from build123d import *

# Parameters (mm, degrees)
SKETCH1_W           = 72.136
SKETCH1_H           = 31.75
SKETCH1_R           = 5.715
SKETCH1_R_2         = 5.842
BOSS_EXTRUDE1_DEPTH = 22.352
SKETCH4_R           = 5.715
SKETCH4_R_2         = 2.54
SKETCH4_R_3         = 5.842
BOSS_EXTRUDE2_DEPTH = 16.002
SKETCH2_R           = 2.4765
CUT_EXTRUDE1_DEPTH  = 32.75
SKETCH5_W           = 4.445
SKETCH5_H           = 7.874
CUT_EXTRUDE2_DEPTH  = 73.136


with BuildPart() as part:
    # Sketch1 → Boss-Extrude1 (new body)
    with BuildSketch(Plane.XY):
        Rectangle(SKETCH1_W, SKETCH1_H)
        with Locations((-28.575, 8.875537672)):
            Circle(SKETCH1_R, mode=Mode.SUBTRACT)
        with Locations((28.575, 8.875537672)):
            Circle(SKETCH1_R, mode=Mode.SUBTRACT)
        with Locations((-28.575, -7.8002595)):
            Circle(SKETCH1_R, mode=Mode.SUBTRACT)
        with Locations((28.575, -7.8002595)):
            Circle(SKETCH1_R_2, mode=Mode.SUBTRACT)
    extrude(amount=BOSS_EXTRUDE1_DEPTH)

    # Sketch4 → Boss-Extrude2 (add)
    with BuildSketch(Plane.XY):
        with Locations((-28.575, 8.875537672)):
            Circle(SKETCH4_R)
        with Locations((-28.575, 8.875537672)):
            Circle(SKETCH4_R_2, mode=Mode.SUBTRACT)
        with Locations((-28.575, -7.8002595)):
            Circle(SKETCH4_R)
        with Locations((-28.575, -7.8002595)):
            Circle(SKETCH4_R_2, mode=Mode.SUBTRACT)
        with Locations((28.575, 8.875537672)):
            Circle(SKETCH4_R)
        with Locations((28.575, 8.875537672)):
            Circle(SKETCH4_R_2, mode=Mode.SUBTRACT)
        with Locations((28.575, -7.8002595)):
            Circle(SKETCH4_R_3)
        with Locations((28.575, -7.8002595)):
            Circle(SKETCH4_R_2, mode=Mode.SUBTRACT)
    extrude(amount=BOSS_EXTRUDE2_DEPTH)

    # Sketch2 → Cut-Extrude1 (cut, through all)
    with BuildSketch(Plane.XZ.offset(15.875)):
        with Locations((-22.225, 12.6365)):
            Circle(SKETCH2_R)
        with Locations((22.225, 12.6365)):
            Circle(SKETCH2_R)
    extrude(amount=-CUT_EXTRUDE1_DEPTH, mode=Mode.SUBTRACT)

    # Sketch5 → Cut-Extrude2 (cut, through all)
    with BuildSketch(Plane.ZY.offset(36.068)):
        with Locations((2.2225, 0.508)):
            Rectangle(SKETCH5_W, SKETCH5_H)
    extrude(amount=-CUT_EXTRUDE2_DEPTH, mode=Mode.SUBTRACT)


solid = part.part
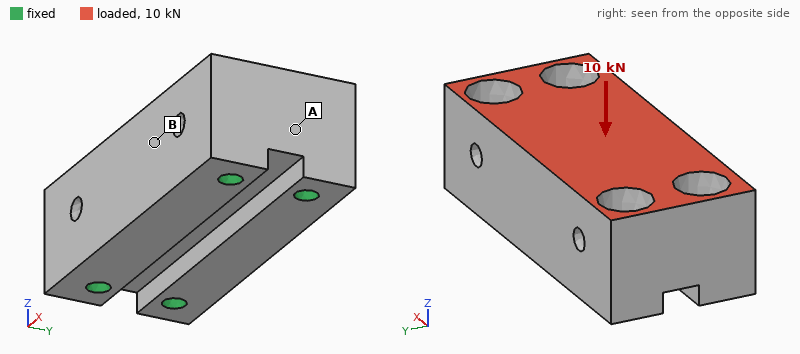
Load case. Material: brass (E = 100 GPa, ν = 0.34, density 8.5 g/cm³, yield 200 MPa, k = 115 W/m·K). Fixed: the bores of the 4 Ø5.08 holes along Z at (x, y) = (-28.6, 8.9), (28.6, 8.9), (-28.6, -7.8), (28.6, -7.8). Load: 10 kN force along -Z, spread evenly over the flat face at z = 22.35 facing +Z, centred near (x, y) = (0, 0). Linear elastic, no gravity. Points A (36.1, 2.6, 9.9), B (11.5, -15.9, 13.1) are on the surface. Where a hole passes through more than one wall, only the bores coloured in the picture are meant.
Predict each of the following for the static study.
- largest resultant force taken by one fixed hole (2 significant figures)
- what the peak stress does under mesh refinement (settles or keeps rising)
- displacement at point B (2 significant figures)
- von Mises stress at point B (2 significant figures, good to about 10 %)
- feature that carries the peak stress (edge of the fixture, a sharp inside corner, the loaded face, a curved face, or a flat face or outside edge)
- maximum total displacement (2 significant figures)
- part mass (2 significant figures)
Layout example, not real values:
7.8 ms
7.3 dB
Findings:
2.8 kN
keeps rising
5.9 µm
11 MPa
edge of the fixture
7.4 µm
370 g
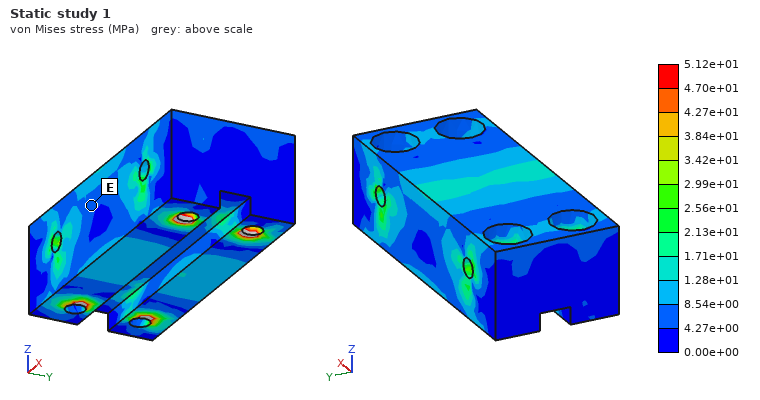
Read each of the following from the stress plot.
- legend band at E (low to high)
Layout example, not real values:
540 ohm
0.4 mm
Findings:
4.27e+00 to 8.54e+00 MPa
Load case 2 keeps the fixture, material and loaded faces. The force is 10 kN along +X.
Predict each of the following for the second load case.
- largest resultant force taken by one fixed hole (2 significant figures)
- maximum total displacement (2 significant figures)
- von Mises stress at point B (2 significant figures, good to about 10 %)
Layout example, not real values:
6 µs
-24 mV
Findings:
2.8 kN
5.7 µm
8.1 MPa
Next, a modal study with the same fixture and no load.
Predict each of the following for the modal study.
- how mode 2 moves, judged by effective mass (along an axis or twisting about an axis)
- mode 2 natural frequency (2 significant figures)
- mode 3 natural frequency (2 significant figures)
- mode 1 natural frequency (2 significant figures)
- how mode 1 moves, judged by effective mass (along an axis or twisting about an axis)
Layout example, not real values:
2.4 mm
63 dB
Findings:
along Y
12 kHz
13 kHz
11 kHz
along Z
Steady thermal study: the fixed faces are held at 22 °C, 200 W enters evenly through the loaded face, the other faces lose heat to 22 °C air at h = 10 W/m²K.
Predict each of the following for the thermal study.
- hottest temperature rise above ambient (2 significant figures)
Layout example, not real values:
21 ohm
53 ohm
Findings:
32 K
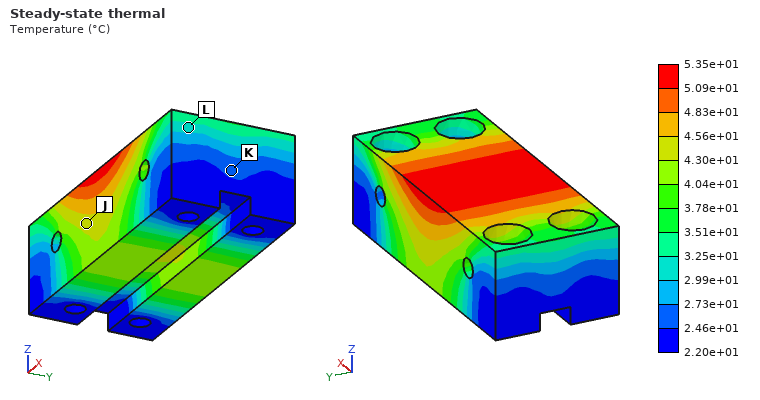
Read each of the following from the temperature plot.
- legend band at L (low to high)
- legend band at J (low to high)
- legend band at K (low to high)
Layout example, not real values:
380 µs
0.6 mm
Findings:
2.99e+01 to 3.25e+01 °C
4.30e+01 to 4.56e+01 °C
2.46e+01 to 2.73e+01 °C
